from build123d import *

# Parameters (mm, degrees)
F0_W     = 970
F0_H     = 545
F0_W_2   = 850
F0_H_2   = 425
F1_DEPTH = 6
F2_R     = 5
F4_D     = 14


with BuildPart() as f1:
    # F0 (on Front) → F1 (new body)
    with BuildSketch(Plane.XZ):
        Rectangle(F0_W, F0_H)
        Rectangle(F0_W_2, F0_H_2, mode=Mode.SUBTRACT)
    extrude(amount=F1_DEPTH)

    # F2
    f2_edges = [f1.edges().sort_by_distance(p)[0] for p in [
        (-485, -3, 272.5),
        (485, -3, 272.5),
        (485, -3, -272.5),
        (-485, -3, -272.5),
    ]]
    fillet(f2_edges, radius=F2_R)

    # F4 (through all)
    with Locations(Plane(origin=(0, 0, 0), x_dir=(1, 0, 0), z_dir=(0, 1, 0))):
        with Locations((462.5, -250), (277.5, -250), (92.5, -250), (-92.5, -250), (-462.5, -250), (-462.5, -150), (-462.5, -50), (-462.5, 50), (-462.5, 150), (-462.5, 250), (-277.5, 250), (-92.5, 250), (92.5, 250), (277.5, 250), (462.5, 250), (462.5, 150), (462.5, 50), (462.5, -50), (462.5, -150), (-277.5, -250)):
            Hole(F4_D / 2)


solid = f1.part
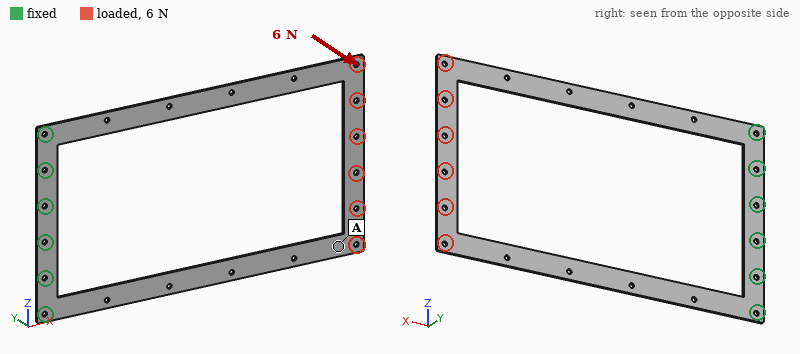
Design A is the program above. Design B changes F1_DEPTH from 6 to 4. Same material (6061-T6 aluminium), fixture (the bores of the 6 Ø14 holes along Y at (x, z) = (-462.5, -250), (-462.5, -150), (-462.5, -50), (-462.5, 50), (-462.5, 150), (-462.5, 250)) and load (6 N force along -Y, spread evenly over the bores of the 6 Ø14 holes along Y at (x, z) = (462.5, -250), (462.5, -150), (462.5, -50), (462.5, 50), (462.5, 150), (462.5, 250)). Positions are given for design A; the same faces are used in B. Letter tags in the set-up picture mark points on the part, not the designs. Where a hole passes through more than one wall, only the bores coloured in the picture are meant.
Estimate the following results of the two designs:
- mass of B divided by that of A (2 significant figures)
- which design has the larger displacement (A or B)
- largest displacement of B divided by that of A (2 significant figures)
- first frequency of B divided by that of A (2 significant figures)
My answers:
0.67
B
3.4
0.67
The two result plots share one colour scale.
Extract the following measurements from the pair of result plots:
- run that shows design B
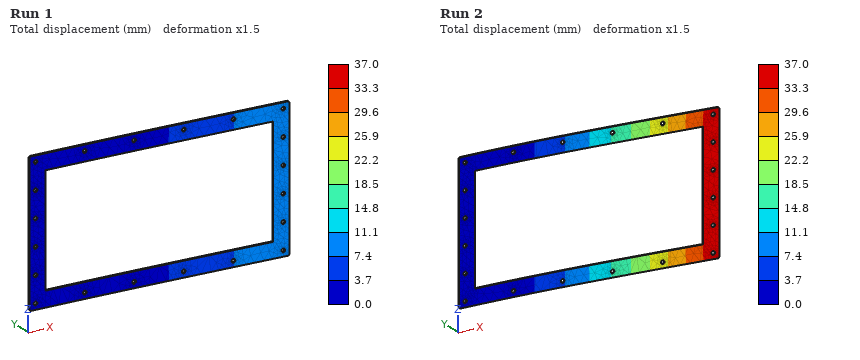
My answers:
Run 2
